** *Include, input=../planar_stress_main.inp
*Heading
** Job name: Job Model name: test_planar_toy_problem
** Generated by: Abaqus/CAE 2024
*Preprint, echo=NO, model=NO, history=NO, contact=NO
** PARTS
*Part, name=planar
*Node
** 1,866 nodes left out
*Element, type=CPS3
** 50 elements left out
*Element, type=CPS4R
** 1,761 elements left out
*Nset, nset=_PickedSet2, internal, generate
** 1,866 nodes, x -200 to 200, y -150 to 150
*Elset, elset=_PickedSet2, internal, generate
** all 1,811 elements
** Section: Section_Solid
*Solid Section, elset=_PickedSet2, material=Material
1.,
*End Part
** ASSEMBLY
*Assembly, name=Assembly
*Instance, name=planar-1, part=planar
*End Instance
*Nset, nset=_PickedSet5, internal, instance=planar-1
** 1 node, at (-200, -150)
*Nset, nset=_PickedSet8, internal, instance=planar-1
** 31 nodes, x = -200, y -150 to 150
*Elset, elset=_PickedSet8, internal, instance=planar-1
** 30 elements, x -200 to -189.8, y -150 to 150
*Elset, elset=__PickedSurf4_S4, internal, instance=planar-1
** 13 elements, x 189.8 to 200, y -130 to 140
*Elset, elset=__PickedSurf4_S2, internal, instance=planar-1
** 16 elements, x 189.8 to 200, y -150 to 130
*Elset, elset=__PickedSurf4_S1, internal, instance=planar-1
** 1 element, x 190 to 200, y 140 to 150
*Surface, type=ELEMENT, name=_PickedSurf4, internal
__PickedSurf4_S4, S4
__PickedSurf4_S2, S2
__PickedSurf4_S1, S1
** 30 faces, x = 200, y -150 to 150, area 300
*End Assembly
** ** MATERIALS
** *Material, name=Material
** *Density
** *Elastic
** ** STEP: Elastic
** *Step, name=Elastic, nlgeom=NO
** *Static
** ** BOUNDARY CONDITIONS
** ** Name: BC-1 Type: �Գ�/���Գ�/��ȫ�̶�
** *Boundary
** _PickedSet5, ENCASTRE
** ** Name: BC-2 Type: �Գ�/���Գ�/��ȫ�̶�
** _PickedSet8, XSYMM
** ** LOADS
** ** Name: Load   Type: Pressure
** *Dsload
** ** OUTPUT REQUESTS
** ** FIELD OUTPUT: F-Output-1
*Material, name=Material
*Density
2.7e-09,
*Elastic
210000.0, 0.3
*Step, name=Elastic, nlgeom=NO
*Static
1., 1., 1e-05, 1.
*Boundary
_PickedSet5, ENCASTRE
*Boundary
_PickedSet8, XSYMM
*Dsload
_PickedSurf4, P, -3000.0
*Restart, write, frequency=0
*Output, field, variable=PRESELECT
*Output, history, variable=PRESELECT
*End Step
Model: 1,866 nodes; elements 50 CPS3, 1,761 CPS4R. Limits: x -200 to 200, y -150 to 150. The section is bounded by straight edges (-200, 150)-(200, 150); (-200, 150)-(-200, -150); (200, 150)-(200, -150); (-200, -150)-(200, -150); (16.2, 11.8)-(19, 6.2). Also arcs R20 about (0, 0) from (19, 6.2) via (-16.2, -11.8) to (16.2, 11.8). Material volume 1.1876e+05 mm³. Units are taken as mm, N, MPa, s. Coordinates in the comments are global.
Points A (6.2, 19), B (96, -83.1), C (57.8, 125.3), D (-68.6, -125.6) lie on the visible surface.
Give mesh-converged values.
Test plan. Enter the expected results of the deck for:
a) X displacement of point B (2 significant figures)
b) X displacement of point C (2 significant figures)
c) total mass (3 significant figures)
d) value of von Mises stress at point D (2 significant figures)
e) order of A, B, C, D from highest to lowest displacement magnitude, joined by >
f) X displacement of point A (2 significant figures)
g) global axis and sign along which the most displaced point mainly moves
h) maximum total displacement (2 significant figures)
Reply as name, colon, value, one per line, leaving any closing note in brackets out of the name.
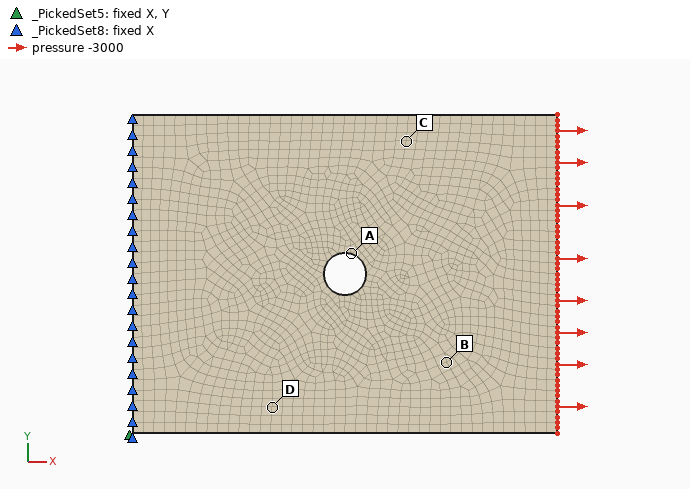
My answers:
X displacement of point B: 4.4 mm
X displacement of point C: 3.8 mm
total mass: 0.321 kg
value of von Mises stress at point D: 3100 MPa
order of A, B, C, D from highest to lowest displacement magnitude, joined by >: B > C > A > D
X displacement of point A: 3.2 mm
global axis and sign along which the most displaced point mainly moves: +X
maximum total displacement: 6.0 mm
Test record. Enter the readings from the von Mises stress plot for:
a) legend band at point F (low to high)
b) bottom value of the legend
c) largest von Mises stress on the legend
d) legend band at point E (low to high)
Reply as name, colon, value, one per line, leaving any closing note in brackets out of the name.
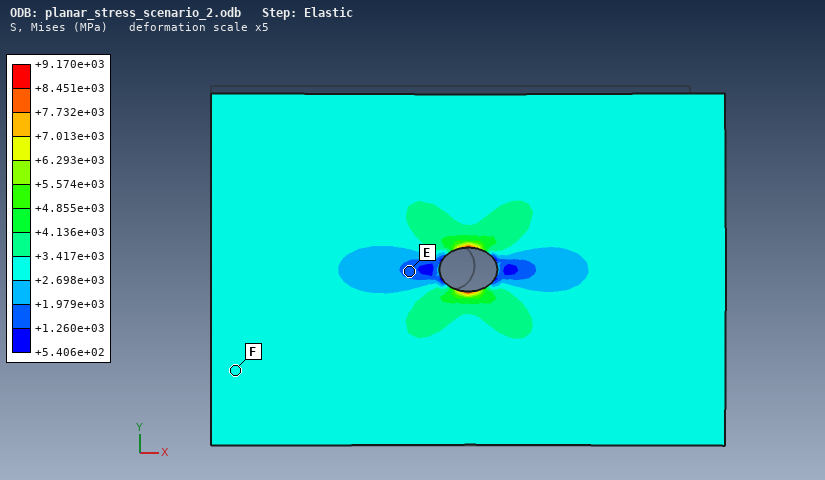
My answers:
legend band at point F: +2.698e+03 to +3.417e+03 MPa
bottom value of the legend: +5.406e+02 MPa
largest von Mises stress on the legend: +9.170e+03 MPa
legend band at point E: +1.260e+03 to +1.979e+03 MPa
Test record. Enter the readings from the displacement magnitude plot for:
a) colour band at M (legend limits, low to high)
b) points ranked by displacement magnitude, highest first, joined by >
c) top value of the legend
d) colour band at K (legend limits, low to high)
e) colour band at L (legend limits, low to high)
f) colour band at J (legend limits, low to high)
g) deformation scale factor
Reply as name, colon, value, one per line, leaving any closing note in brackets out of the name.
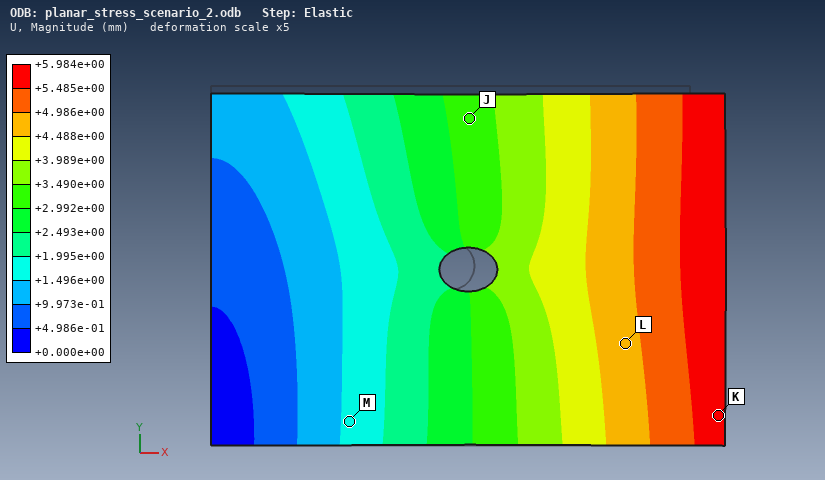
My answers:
colour band at M: +1.496e+00 to +1.995e+00 mm
points ranked by displacement magnitude, highest first, joined by >: K > L > J > M
top value of the legend: +5.984e+00 mm
colour band at K: +5.485e+00 to +5.984e+00 mm
colour band at L: +4.488e+00 to +4.986e+00 mm
colour band at J: +2.992e+00 to +3.490e+00 mm
deformation scale factor: 5
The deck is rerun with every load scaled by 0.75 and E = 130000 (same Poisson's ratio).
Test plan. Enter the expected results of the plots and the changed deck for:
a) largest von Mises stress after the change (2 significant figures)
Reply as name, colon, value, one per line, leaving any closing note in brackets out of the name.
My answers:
largest von Mises stress after the change: 6900 MPa
